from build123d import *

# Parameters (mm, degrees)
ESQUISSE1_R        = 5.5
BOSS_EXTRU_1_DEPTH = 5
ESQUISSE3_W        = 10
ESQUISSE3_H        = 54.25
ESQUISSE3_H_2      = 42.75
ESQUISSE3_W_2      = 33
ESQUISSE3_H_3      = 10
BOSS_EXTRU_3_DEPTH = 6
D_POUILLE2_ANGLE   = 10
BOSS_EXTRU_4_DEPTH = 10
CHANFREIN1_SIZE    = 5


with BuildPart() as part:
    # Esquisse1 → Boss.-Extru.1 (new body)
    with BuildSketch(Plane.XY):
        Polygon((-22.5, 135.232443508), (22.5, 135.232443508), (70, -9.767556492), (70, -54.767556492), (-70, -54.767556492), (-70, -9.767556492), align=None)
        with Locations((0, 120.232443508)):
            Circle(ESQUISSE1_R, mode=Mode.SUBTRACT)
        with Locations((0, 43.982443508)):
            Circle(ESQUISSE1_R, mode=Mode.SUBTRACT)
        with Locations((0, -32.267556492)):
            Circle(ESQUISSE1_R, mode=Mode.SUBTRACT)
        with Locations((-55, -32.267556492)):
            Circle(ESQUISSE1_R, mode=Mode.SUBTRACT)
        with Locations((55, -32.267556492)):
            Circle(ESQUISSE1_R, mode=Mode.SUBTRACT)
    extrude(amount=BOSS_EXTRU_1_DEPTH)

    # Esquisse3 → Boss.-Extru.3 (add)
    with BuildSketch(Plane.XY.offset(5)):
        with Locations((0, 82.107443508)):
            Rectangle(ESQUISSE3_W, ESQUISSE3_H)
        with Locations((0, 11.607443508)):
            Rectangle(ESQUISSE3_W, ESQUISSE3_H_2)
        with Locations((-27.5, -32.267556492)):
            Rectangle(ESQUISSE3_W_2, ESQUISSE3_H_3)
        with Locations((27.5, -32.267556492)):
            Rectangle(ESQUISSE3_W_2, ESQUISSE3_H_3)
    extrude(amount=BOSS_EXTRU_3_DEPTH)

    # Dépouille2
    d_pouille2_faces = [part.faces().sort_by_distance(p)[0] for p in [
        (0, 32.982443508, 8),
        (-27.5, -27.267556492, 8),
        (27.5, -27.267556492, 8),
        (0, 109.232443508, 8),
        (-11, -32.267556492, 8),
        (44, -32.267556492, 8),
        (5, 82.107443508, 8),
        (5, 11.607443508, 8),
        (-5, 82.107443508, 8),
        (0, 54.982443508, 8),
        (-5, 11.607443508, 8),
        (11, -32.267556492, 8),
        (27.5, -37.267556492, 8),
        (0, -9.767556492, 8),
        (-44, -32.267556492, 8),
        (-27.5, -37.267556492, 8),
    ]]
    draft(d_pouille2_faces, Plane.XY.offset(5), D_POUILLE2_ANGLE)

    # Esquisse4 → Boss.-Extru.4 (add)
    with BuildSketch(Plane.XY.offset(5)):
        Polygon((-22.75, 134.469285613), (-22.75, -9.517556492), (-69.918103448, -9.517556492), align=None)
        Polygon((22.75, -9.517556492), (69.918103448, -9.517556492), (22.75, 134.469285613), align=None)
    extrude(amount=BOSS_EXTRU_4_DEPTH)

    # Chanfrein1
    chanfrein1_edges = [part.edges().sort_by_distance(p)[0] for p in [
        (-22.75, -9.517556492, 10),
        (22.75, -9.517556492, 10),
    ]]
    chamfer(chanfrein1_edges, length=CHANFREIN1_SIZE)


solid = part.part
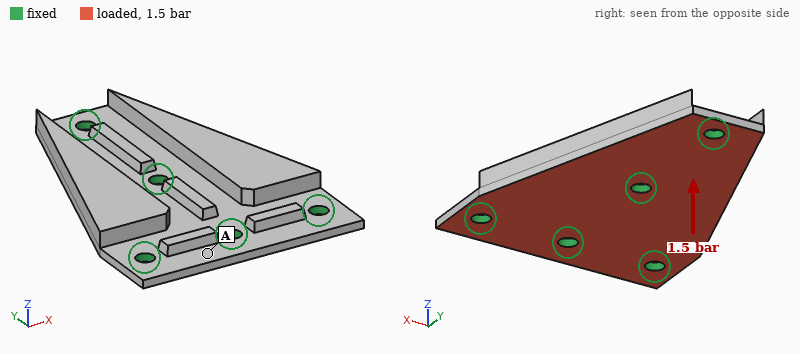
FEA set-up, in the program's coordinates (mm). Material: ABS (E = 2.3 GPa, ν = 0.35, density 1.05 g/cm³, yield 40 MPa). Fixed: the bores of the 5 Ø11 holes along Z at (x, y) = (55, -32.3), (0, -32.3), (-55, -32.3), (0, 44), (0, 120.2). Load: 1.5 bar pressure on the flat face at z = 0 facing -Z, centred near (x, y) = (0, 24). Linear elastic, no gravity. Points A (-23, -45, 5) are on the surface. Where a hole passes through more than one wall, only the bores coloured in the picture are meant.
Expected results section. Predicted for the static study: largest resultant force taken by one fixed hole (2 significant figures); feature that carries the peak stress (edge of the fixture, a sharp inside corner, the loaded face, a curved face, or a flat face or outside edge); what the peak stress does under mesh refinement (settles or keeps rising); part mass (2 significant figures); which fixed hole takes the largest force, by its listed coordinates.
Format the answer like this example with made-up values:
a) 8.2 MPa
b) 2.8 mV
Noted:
a) 920 N
b) edge of the fixture
c) keeps rising
d) 180 g
e) (0, 44)
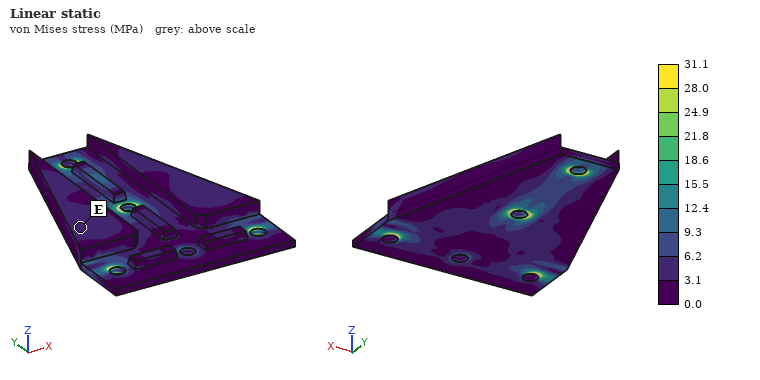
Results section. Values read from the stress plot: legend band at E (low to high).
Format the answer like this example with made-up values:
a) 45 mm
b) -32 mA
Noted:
a) 3.1 to 6.2 MPa
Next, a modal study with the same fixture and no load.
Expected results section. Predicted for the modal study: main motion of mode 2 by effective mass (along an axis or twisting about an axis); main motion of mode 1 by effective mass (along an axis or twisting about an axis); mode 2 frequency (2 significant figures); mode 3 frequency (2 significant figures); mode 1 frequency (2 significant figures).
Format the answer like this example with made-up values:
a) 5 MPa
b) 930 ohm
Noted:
a) along Z
b) twisting about Y
c) 650 Hz
d) 1300 Hz
e) 590 Hz
